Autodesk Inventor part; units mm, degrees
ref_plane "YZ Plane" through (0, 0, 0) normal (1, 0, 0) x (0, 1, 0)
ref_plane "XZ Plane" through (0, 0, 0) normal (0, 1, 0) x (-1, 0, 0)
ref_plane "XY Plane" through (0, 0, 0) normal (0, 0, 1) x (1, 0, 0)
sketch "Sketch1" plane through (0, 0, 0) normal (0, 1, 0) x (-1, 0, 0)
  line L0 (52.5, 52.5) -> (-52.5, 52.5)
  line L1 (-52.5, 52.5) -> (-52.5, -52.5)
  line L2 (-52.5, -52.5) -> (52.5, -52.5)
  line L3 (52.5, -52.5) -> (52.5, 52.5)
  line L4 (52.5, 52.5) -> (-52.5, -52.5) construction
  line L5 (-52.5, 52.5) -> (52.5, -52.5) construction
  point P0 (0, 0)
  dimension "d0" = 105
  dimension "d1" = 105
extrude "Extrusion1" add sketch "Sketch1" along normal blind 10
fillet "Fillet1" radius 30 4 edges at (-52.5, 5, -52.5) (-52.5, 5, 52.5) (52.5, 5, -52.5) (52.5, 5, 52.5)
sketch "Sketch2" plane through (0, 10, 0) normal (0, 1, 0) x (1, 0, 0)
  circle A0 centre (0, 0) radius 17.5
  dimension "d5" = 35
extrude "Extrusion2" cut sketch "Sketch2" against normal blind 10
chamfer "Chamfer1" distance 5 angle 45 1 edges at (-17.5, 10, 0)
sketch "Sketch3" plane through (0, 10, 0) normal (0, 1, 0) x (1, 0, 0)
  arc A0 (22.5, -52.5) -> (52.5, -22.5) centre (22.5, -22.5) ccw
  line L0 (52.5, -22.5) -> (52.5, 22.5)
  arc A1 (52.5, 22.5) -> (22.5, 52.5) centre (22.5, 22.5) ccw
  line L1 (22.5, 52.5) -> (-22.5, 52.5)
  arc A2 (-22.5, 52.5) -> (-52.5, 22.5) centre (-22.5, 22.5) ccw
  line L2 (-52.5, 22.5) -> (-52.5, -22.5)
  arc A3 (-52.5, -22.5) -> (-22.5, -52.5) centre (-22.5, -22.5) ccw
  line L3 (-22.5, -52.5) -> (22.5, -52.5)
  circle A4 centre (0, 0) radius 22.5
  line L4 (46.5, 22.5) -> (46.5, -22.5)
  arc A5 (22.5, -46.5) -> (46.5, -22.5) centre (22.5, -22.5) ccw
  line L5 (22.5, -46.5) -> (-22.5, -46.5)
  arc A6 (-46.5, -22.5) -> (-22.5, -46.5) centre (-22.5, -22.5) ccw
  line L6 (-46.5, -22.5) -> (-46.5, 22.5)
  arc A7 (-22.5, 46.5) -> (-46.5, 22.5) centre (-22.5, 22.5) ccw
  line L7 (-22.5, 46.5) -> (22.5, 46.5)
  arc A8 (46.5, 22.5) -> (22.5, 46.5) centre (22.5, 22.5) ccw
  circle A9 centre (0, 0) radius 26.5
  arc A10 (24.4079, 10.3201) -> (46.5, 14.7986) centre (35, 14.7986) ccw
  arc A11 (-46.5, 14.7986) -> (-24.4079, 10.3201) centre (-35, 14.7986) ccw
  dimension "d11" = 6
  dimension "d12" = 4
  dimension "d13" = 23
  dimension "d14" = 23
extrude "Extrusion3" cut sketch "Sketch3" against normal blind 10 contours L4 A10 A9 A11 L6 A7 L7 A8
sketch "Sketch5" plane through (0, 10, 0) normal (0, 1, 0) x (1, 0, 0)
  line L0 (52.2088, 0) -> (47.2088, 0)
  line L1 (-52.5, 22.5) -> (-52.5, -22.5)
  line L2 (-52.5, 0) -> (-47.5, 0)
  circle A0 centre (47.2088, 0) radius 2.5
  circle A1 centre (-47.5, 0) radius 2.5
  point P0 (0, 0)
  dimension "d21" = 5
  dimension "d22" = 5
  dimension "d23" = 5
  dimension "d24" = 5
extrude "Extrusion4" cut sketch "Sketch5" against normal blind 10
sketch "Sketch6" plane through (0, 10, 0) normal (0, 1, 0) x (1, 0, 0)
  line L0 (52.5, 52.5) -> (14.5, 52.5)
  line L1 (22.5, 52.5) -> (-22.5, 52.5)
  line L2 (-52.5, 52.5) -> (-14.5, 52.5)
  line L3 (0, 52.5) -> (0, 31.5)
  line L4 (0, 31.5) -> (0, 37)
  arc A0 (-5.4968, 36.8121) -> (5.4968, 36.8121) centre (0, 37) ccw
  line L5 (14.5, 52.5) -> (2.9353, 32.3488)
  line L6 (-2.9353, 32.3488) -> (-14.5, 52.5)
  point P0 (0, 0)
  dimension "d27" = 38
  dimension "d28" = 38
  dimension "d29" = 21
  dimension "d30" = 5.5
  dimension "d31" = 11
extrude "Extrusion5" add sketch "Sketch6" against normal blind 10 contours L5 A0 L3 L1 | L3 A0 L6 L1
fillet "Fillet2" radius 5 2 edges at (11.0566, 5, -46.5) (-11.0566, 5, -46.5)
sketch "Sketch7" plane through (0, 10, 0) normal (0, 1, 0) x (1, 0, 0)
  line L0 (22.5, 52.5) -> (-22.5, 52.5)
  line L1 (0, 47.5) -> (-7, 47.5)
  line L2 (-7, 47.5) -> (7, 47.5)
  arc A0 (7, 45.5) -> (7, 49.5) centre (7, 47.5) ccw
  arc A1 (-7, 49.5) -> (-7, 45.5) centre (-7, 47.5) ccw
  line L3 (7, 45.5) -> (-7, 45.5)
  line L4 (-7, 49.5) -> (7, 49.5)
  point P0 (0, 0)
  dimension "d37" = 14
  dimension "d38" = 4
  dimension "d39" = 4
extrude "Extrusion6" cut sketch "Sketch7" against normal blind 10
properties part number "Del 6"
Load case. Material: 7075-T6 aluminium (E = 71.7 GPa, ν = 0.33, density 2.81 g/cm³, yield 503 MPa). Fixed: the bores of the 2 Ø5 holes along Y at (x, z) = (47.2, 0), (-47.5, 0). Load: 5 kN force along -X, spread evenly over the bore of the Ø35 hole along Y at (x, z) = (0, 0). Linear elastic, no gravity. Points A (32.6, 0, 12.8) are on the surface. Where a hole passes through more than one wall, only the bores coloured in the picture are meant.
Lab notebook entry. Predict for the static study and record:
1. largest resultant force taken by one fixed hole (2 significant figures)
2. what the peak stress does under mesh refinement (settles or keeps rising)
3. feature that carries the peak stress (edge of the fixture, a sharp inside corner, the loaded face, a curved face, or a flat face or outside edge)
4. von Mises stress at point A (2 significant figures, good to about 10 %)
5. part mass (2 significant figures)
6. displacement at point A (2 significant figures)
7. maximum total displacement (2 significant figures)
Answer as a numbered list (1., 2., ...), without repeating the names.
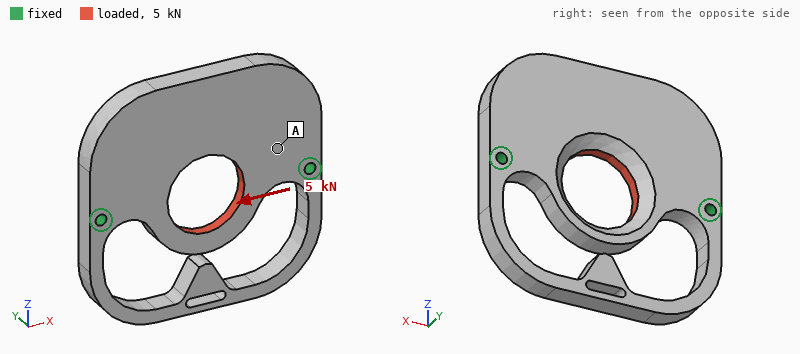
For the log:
1. 2.5 kN
2. keeps rising
3. edge of the fixture
4. 6.6 MPa
5. 180 g
6. 5.0 µm
7. 25 µm
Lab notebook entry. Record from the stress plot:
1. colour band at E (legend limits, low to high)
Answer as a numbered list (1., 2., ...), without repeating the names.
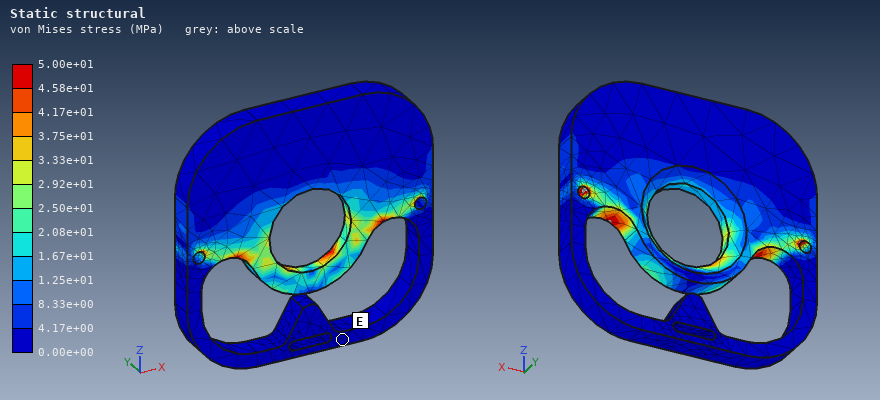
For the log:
1. 0.00e+00 to 4.17e+00 MPa
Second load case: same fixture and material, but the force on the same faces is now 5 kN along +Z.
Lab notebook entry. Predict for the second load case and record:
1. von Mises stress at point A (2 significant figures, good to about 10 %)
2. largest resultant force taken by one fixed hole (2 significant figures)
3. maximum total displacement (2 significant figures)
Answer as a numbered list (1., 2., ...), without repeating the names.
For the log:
1. 19 MPa
2. 2.7 kN
3. 61 µm
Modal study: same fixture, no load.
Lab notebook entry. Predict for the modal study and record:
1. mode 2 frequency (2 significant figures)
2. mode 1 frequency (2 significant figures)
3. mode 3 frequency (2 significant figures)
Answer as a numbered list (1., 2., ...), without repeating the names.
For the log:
1. 1800 Hz
2. 1400 Hz
3. 1800 Hz
